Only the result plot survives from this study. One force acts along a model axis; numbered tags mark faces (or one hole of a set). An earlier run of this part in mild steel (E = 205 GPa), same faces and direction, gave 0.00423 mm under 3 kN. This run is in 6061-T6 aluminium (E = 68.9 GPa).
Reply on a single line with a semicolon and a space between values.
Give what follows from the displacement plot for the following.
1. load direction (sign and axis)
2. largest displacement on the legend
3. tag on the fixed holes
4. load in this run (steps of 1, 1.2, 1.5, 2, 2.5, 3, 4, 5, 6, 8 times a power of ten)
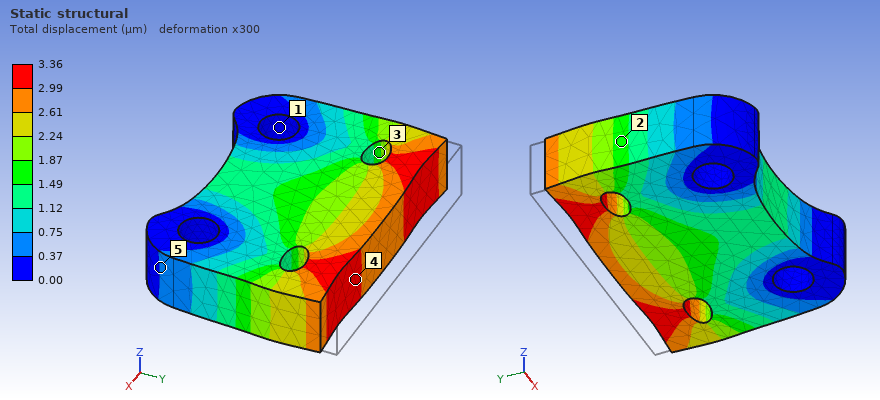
-Y; 3.36 µm; 1; 800 N
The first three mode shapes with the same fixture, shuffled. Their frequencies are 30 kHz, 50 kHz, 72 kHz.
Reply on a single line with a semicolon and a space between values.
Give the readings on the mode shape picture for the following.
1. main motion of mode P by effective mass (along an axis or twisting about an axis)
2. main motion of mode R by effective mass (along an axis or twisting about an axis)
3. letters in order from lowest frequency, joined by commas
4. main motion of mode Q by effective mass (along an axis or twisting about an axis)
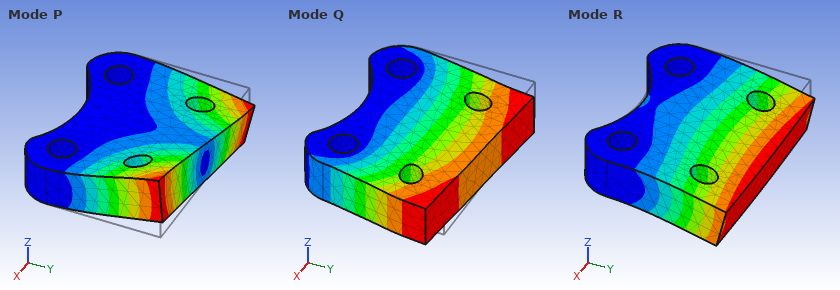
twisting about Y; along Z; R, P, Q; along X
